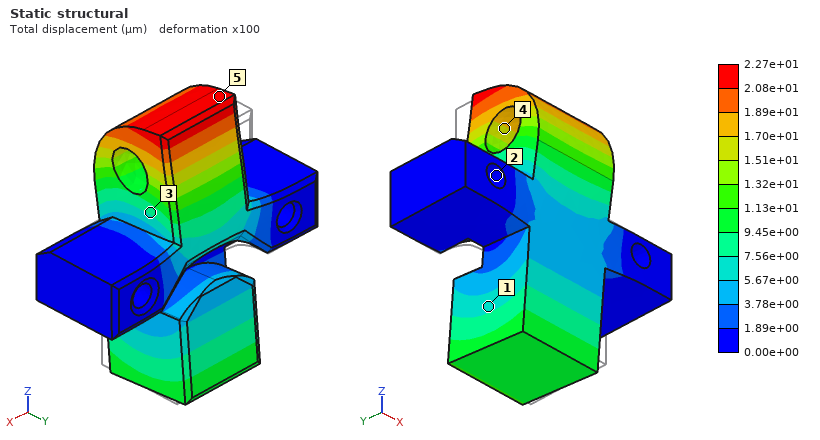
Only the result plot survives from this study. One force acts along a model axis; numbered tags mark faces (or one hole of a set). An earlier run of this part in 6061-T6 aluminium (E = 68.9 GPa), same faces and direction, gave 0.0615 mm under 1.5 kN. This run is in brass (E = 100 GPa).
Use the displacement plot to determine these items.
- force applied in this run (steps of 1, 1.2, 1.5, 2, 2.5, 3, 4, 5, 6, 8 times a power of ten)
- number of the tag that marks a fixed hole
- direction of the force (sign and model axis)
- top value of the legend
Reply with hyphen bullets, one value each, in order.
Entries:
- 800 N
- 2
- -Y
- 2.27e+01 µm
